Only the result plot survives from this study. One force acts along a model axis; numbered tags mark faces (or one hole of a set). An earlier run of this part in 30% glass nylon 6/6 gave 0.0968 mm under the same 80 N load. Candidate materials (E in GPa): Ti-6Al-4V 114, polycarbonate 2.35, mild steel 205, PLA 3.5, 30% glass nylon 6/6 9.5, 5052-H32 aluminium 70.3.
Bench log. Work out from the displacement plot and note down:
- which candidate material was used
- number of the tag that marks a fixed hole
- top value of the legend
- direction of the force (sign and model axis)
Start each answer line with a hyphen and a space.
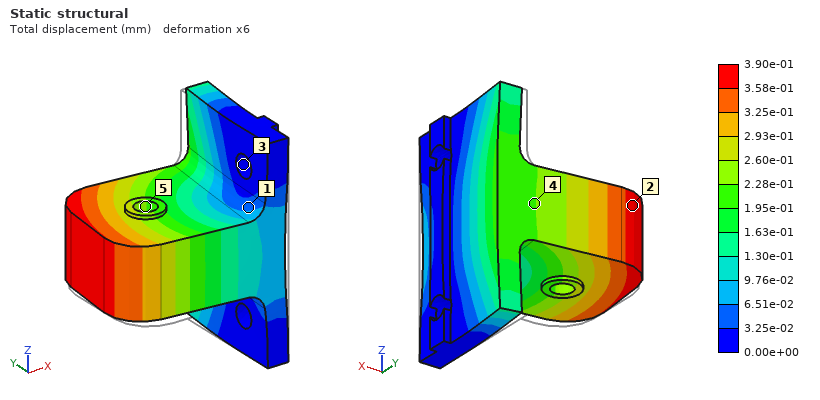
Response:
- polycarbonate
- 3
- 3.90e-01 mm
- +Y
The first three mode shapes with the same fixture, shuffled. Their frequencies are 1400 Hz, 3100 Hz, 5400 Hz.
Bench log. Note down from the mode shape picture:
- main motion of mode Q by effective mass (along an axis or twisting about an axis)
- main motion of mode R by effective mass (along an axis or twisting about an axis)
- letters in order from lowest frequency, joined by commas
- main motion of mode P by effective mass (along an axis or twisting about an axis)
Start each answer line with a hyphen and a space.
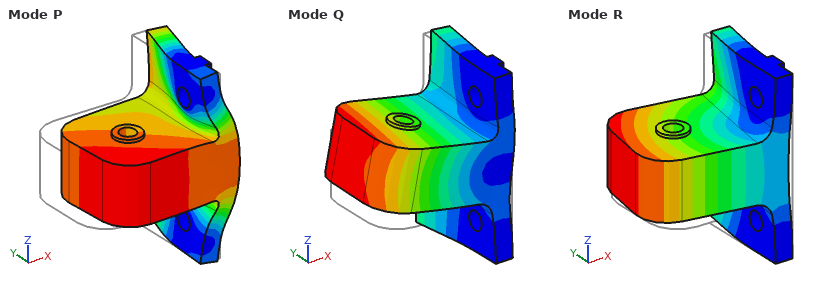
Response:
- along Z
- along Y
- R, Q, P
- along X
